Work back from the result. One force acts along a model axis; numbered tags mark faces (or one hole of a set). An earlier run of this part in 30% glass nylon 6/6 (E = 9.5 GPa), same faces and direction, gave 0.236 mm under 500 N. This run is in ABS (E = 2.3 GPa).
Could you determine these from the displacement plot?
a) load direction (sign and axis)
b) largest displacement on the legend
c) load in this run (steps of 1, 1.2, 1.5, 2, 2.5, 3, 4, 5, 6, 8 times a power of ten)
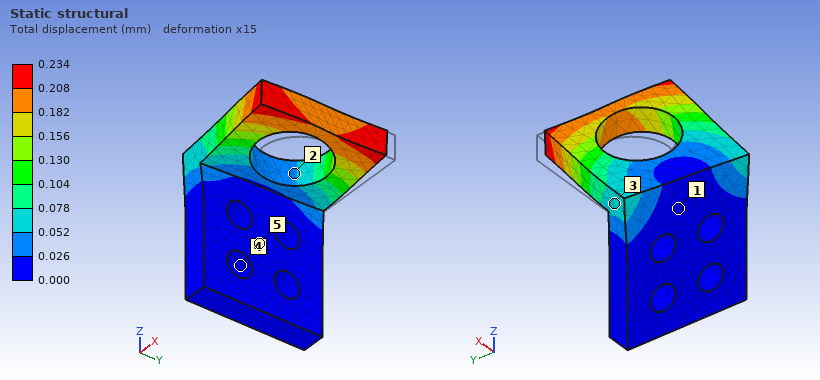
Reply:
-Y
0.234 mm
120 N
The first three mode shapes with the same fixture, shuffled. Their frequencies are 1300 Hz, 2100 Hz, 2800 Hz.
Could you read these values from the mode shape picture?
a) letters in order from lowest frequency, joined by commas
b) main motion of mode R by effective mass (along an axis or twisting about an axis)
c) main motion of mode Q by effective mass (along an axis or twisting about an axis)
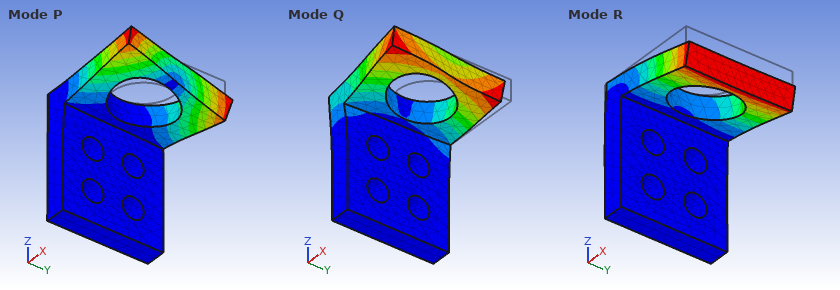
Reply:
R, Q, P
along Z
along Y
